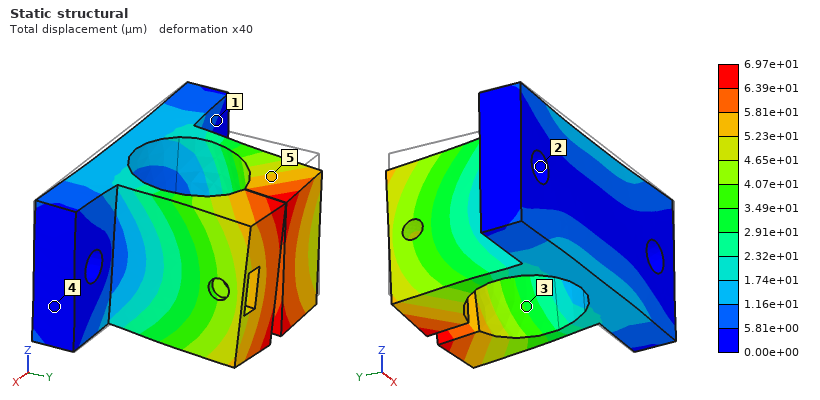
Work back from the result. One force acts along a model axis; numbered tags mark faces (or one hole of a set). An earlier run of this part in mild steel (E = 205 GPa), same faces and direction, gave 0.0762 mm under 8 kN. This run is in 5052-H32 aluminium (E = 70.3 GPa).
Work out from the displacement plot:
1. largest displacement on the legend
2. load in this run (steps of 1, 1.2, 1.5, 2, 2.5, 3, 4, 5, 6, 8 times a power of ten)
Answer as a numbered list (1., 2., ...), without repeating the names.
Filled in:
1. 6.97e+01 µm
2. 2.5 kN
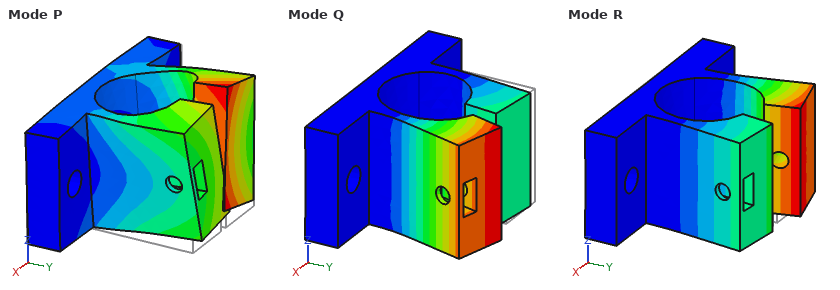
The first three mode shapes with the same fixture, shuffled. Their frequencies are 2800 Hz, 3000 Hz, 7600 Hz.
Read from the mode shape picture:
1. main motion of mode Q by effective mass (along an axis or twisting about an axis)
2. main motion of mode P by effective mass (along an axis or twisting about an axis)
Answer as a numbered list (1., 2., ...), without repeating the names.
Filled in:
1. along X
2. along Z
